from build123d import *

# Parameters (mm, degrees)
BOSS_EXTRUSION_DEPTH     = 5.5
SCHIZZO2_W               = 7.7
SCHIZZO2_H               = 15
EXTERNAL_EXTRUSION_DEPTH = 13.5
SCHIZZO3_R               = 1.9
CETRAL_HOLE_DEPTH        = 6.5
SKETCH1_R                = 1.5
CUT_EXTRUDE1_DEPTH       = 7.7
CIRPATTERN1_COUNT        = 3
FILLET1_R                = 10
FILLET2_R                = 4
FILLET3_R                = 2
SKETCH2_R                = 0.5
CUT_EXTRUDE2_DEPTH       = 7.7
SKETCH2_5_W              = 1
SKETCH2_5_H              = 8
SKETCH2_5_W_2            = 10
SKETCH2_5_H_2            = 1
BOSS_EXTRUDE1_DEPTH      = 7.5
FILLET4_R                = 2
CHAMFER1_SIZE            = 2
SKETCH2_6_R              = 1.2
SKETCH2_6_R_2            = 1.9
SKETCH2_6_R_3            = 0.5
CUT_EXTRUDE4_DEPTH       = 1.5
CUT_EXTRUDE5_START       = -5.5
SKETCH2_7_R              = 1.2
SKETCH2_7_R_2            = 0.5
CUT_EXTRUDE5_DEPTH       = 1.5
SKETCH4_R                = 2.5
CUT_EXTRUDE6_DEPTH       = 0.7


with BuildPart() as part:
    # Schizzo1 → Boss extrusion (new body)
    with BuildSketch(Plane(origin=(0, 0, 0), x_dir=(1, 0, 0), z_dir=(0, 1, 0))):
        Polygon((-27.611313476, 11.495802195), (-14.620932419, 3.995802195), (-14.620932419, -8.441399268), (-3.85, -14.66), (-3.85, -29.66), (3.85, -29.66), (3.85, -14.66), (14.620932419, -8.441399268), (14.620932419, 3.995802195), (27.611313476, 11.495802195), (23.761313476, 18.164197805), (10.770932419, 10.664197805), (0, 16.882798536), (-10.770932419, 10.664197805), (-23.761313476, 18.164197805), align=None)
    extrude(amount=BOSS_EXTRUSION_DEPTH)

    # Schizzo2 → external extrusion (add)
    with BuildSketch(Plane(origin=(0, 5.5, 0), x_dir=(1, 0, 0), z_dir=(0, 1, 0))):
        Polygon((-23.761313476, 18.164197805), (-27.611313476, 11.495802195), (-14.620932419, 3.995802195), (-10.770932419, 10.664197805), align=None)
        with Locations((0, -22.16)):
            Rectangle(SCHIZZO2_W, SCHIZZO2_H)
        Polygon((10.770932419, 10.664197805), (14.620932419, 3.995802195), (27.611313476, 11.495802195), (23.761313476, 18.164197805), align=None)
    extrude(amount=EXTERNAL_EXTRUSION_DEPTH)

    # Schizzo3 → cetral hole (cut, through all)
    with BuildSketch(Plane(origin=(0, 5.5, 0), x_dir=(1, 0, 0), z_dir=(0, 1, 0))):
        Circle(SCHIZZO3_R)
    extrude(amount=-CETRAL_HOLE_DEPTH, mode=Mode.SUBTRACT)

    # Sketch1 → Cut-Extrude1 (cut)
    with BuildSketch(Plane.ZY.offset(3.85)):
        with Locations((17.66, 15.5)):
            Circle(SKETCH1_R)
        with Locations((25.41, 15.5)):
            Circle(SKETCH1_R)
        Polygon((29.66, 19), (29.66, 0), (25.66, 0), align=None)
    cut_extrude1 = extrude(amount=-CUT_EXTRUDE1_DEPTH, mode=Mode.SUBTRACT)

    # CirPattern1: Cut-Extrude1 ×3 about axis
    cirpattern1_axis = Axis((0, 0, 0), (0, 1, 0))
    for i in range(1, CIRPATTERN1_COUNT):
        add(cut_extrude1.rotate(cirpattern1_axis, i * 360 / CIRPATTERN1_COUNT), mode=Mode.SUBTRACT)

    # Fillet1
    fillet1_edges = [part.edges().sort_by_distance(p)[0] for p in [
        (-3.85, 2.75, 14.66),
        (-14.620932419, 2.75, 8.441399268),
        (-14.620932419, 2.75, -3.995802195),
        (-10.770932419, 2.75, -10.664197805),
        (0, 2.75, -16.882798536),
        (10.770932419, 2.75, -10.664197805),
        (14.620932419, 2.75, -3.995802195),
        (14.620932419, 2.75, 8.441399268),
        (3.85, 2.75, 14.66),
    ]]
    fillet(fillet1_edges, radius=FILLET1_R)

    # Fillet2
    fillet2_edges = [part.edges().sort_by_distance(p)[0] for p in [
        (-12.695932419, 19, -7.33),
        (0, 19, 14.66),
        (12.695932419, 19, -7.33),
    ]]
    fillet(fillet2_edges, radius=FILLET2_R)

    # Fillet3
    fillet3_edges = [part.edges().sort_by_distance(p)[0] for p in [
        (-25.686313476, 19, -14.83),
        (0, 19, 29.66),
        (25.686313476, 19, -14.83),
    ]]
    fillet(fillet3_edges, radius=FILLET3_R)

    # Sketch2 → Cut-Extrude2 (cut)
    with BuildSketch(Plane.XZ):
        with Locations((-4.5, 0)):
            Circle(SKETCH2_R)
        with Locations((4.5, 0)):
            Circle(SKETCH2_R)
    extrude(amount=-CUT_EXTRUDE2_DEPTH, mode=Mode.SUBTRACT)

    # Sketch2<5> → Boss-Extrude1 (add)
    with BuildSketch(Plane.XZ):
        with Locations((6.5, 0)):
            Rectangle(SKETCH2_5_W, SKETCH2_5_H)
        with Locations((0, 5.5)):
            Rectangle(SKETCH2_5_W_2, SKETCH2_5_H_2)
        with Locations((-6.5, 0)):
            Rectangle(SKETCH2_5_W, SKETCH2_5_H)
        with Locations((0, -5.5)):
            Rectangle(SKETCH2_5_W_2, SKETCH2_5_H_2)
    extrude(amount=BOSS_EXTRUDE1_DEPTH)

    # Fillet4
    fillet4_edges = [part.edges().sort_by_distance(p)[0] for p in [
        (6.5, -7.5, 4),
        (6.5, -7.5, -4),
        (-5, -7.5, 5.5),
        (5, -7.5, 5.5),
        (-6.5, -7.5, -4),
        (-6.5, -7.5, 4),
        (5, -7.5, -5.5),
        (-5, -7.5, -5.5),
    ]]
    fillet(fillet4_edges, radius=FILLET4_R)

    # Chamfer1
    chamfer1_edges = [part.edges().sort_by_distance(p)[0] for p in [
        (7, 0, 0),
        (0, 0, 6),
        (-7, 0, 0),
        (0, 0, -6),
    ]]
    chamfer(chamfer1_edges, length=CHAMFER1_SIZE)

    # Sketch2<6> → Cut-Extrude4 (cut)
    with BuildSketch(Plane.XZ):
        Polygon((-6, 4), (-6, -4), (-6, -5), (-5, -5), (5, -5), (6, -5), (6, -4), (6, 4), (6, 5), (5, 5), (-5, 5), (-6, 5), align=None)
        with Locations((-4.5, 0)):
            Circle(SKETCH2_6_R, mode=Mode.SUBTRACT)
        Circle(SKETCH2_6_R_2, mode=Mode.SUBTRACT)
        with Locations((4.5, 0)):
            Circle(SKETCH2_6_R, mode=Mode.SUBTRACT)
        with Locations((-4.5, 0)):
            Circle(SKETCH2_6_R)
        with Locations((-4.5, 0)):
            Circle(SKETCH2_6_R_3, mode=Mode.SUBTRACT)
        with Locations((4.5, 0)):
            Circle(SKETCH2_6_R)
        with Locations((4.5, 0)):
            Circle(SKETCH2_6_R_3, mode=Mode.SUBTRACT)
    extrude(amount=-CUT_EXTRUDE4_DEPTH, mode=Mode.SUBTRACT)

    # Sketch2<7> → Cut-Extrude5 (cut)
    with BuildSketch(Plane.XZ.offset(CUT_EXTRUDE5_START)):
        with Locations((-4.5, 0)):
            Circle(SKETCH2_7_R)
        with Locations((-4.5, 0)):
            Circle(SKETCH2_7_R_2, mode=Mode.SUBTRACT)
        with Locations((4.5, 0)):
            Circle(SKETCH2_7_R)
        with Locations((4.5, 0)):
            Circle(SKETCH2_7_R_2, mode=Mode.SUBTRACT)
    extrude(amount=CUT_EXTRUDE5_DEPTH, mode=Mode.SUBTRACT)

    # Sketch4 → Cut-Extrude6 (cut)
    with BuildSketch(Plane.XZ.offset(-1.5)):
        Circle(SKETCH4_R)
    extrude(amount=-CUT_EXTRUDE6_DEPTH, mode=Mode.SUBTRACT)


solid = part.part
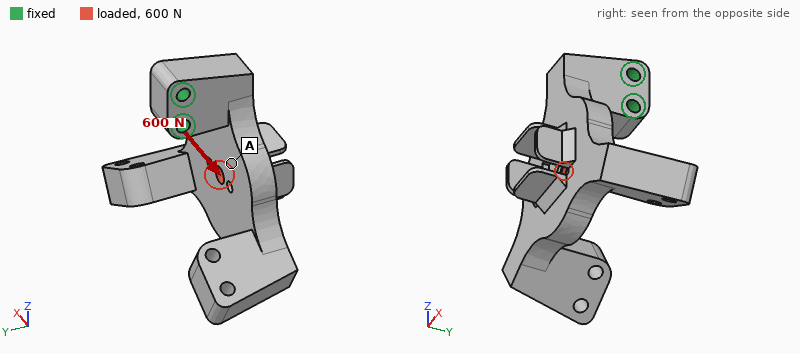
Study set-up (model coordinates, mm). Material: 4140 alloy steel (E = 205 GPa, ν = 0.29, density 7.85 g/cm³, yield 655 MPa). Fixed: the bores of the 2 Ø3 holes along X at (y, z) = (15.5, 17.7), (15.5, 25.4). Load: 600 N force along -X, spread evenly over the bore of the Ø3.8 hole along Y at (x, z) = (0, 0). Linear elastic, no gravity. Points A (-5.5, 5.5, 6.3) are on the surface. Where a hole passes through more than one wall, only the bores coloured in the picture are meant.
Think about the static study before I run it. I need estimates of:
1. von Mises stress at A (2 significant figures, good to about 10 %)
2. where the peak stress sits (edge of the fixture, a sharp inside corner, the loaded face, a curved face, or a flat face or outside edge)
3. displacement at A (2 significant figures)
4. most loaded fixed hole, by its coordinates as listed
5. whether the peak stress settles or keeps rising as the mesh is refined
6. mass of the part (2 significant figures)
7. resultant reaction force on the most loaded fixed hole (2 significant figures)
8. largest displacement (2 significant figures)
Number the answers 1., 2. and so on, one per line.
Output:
1. 17 MPa
2. edge of the fixture
3. 33 µm
4. (15.5, 17.7)
5. keeps rising
6. 74 g
7. 1.3 kN
8. 95 µm
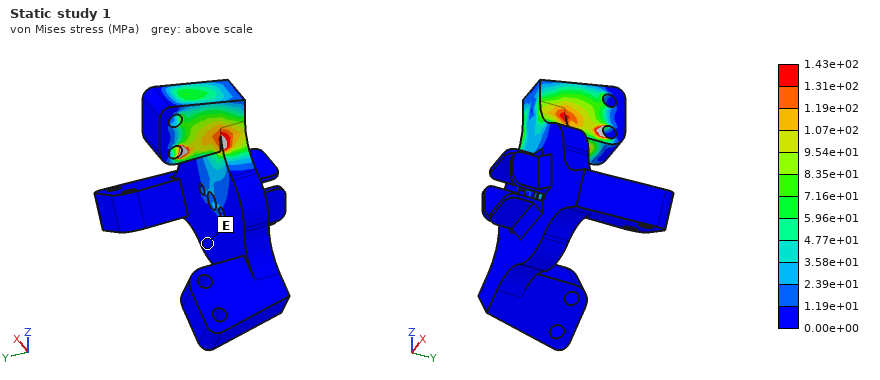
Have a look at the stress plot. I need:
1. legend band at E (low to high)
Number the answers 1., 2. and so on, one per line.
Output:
1. 0.00e+00 to 1.19e+01 MPa
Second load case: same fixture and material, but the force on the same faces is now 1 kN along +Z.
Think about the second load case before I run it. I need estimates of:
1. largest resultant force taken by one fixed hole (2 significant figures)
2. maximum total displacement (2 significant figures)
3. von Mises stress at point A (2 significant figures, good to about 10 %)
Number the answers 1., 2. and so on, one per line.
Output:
1. 1.3 kN
2. 6.0 µm
3. 17 MPa
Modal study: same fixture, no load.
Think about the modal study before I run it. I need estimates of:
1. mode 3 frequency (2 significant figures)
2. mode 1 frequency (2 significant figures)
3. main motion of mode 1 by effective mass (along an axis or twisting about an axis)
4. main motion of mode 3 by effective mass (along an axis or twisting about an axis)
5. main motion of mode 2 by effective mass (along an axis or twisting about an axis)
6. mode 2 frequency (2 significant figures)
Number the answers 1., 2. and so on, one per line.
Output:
1. 2000 Hz
2. 1500 Hz
3. along Y
4. twisting about Z
5. along X
6. 1600 Hz
